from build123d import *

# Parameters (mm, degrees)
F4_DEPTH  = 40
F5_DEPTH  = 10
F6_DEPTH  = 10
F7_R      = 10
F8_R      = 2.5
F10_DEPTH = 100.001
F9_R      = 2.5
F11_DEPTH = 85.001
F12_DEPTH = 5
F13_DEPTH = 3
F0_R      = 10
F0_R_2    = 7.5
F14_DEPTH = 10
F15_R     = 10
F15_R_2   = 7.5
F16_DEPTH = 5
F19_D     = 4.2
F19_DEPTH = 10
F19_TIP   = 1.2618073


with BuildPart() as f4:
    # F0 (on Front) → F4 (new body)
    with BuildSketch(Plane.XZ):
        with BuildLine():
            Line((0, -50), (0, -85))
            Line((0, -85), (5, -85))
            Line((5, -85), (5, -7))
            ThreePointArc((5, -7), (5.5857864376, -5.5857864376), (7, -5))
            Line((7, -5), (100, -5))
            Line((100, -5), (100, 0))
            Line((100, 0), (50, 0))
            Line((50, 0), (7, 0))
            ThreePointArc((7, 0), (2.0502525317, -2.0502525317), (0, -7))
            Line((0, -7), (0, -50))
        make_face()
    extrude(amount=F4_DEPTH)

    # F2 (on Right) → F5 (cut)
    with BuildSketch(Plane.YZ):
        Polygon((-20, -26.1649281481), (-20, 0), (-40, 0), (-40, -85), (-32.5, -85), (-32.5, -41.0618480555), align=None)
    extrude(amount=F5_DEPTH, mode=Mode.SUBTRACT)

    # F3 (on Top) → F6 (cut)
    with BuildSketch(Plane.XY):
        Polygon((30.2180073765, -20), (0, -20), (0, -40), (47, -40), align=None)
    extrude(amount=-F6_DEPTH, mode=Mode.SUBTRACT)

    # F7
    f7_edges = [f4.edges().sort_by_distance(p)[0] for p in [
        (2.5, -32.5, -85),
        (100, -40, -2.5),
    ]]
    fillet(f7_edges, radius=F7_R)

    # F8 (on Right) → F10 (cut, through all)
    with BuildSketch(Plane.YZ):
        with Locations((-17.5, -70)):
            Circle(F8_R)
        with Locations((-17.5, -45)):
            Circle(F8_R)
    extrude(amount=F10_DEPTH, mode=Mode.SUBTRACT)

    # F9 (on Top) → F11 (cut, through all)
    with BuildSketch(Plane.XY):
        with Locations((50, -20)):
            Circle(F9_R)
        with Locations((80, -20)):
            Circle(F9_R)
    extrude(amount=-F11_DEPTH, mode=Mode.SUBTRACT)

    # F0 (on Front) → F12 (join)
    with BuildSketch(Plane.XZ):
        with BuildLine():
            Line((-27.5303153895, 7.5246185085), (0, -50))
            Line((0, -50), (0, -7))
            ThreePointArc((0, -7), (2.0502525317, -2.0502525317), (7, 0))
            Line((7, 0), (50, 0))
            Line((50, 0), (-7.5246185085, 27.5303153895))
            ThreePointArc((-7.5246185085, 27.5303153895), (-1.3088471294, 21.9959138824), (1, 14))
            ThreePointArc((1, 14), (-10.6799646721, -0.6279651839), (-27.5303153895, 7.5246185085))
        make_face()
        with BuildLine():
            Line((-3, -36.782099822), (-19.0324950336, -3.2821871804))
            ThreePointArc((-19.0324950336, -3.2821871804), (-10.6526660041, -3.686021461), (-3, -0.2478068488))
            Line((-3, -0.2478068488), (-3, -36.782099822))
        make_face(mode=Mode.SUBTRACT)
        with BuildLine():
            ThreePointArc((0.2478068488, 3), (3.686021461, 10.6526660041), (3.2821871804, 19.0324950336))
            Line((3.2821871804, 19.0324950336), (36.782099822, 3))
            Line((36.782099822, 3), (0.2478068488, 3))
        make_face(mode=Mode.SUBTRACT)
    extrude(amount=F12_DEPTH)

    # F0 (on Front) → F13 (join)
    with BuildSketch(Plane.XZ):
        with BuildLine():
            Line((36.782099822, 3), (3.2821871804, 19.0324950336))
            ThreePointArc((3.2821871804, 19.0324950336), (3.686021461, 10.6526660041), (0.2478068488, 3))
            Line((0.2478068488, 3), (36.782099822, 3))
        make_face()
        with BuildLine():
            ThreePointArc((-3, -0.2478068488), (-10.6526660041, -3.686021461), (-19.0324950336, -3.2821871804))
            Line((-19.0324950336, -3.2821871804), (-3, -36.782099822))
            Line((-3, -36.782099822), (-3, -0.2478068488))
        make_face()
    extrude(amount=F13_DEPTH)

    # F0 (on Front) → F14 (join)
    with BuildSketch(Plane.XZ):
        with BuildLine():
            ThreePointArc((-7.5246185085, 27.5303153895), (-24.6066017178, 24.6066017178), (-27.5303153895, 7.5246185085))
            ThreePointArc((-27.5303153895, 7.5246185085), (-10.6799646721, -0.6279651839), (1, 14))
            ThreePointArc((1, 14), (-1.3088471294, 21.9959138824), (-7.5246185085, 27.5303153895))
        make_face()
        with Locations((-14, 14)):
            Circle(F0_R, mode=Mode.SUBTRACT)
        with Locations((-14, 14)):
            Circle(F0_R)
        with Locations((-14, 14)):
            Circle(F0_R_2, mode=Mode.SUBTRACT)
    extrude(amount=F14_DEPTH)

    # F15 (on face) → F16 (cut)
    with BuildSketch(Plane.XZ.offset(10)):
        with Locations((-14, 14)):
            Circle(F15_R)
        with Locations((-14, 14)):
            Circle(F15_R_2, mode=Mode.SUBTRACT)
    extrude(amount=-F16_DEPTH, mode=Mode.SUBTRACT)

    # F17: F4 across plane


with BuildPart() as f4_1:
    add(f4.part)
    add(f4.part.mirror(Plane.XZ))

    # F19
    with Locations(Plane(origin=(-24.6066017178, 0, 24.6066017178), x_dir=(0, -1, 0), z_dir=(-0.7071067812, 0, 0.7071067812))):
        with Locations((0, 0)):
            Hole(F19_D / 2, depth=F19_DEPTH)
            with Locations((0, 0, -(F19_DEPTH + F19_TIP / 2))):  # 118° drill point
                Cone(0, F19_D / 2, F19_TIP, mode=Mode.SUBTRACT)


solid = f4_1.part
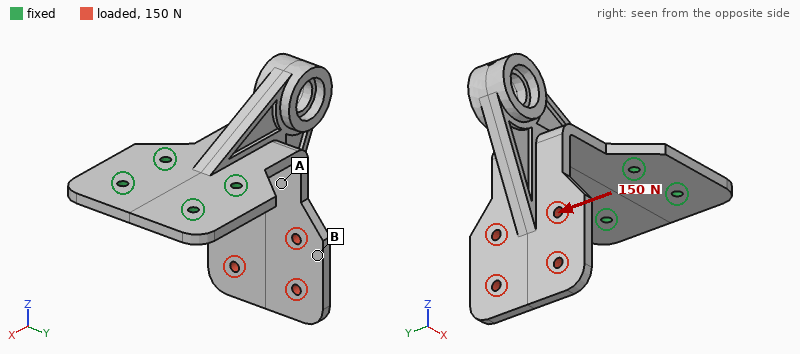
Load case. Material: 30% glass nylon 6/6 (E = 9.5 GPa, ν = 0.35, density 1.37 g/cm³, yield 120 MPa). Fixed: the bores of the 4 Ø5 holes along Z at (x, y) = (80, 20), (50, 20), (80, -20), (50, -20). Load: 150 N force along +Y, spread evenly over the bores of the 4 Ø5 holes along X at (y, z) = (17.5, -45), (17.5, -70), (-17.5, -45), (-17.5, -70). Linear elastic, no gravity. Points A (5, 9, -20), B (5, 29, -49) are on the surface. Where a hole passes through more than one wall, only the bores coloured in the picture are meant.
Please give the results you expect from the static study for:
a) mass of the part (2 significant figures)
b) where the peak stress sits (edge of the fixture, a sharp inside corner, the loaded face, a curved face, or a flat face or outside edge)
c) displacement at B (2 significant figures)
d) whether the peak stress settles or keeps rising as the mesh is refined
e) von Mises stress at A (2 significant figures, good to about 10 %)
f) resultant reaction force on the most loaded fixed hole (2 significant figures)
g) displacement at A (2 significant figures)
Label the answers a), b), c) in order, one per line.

a) 99 g
b) edge of the fixture
c) 1.4 mm
d) keeps rising
e) 4.8 MPa
f) 290 N
g) 0.53 mm
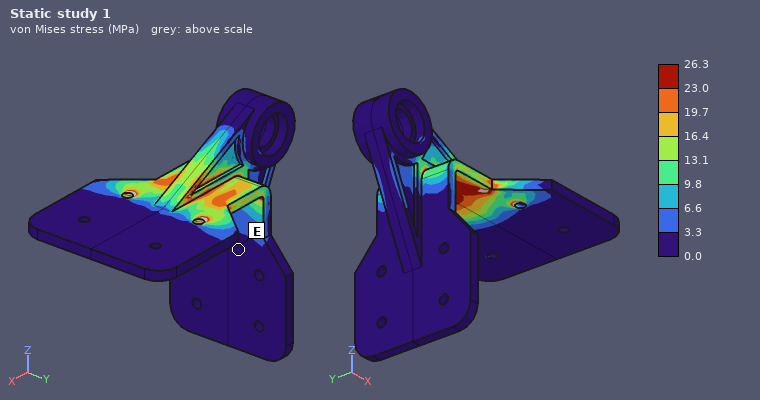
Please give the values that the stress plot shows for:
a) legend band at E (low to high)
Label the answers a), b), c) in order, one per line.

a) 0.0 to 3.3 MPa
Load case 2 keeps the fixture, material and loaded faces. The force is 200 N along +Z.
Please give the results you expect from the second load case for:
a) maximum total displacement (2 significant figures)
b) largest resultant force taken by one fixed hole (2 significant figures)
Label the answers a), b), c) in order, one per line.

a) 1.9 mm
b) 170 N
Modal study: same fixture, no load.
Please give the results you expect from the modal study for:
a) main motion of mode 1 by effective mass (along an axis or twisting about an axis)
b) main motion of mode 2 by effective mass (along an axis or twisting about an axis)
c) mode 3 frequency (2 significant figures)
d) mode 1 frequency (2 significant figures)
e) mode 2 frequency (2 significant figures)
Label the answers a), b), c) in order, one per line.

a) along Z
b) along Y
c) 760 Hz
d) 210 Hz
e) 300 Hz
